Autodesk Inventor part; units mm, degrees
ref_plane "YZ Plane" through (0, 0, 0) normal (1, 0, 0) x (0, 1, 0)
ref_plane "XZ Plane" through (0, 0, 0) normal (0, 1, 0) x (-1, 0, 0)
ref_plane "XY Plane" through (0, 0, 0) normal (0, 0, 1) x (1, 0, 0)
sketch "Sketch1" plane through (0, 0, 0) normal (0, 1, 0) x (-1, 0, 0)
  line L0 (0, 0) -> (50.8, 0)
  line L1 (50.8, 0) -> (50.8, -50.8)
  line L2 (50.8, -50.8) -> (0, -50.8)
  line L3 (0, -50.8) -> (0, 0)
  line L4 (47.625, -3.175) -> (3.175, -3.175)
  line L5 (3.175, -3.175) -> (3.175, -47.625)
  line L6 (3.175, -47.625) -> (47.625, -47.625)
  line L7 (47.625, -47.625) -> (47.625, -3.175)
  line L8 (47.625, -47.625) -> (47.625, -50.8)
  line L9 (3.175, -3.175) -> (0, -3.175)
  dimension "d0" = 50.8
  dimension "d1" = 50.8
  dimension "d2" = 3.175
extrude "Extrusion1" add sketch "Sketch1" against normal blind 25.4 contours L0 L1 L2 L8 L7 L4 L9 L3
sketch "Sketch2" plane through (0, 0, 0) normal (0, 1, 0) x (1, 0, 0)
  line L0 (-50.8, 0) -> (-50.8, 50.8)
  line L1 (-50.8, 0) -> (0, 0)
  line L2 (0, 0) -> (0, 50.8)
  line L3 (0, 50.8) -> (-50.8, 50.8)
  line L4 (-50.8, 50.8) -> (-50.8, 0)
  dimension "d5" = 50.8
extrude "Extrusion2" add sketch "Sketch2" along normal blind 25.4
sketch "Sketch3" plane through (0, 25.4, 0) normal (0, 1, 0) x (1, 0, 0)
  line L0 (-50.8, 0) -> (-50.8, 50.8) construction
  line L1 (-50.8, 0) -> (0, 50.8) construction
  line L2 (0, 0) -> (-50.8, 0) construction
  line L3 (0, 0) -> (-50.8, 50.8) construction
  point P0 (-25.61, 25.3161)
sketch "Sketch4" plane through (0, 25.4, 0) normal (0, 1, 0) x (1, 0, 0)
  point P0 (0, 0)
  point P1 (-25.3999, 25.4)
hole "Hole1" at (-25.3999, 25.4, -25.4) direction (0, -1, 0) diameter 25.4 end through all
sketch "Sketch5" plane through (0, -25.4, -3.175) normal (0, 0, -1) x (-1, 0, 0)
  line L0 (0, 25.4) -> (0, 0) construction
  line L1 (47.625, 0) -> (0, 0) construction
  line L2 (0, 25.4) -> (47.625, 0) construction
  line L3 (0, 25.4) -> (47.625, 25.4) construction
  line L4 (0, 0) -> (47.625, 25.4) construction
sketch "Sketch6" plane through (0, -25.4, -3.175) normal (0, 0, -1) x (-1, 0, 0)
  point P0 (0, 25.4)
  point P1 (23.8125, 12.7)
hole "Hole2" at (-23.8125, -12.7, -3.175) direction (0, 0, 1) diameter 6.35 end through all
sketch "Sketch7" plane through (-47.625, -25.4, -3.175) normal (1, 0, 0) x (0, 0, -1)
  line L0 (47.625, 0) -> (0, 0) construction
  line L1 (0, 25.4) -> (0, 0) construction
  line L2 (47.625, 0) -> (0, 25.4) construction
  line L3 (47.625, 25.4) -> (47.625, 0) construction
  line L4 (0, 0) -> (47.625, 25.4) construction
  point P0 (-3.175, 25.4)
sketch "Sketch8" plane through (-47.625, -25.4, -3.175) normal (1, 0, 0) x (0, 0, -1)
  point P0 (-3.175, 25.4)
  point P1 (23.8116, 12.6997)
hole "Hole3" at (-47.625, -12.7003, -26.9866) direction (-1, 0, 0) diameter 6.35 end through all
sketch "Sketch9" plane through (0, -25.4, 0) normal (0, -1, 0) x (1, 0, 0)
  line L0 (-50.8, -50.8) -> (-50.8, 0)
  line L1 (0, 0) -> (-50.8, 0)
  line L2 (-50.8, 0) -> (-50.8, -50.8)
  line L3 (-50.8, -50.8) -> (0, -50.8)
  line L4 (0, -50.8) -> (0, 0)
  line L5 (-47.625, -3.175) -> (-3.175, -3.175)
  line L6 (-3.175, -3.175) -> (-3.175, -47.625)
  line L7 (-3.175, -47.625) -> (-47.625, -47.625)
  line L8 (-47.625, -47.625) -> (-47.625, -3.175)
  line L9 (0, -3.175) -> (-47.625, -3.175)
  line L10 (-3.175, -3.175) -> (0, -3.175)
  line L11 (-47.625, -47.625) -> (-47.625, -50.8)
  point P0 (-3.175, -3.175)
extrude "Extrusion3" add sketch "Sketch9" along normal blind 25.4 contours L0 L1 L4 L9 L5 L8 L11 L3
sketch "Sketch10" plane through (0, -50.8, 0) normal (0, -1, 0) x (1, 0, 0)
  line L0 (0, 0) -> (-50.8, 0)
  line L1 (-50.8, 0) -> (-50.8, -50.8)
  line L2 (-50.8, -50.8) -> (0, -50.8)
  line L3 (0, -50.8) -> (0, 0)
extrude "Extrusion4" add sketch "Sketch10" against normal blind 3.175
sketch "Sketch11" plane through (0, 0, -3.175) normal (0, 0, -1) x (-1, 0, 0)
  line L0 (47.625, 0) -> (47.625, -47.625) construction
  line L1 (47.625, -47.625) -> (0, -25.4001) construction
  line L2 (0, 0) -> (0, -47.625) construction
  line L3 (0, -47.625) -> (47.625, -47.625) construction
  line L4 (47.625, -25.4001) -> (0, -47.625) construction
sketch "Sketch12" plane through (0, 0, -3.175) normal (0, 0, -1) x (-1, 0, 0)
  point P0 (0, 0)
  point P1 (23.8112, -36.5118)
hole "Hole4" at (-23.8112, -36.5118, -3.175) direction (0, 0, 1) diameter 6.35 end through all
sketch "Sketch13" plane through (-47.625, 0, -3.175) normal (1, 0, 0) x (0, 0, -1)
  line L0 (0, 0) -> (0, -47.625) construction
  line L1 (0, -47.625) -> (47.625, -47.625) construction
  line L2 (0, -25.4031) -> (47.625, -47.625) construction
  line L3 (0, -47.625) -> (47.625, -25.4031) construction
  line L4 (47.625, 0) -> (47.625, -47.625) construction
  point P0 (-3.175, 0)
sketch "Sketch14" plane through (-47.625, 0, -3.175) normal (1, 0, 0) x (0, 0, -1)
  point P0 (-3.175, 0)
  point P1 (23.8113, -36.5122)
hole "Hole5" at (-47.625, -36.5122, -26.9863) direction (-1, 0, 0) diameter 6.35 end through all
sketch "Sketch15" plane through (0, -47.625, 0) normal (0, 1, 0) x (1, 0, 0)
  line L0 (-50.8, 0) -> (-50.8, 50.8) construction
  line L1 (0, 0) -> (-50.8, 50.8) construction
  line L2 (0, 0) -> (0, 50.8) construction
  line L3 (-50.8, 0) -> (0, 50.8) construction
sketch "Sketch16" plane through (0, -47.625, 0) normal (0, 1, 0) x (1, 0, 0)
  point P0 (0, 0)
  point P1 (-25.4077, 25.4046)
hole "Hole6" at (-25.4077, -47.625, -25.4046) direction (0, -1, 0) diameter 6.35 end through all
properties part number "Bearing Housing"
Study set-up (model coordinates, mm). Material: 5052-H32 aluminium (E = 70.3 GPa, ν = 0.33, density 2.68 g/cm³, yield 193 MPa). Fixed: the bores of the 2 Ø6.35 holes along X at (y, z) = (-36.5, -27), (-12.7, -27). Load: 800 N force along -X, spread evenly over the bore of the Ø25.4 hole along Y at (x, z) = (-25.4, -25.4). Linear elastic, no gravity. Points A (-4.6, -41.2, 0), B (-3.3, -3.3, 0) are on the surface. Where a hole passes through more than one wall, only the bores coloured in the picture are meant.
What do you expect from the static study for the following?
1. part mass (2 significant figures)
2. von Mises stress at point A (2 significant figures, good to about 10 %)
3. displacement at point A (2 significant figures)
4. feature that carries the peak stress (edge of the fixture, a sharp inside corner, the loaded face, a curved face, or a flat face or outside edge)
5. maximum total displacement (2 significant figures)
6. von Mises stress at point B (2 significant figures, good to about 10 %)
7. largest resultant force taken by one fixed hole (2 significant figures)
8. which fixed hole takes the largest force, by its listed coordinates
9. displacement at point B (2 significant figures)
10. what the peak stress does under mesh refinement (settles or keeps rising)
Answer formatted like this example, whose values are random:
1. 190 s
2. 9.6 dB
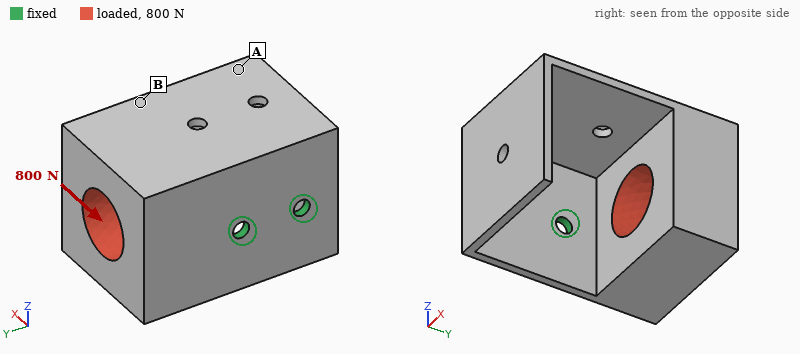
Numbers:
1. 200 g
2. 17 MPa
3. 0.21 mm
4. edge of the fixture
5. 0.35 mm
6. 35 MPa
7. 1.2 kN
8. (-12.7, -27)
9. 0.25 mm
10. keeps rising
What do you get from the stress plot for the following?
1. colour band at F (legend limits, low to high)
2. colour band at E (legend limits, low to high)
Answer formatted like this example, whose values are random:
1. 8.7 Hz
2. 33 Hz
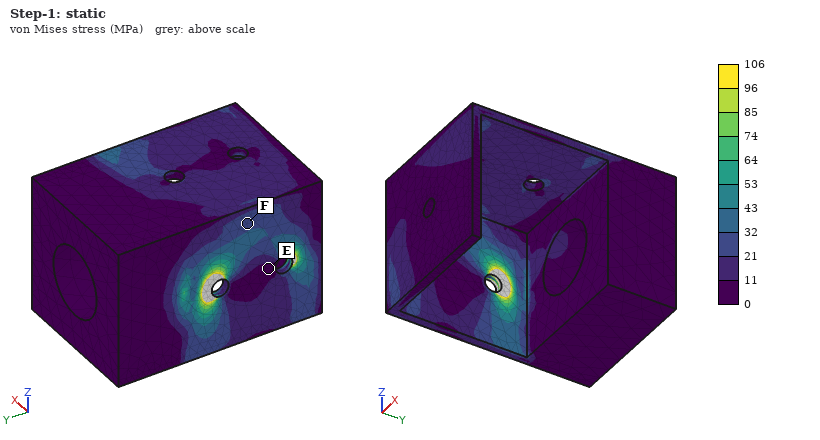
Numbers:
1. 21 to 32 MPa
2. 0 to 11 MPa
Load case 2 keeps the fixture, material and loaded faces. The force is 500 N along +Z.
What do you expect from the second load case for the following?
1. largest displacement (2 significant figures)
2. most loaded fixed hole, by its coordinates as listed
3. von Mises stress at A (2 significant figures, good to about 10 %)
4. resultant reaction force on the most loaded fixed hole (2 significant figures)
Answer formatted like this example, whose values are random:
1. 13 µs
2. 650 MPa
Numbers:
1. 0.32 mm
2. (-12.7, -27)
3. 11 MPa
4. 900 N
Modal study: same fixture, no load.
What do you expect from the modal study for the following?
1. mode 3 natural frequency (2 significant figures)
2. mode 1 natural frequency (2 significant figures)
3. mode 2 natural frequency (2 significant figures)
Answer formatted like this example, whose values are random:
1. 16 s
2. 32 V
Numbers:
1. 1700 Hz
2. 520 Hz
3. 720 Hz
